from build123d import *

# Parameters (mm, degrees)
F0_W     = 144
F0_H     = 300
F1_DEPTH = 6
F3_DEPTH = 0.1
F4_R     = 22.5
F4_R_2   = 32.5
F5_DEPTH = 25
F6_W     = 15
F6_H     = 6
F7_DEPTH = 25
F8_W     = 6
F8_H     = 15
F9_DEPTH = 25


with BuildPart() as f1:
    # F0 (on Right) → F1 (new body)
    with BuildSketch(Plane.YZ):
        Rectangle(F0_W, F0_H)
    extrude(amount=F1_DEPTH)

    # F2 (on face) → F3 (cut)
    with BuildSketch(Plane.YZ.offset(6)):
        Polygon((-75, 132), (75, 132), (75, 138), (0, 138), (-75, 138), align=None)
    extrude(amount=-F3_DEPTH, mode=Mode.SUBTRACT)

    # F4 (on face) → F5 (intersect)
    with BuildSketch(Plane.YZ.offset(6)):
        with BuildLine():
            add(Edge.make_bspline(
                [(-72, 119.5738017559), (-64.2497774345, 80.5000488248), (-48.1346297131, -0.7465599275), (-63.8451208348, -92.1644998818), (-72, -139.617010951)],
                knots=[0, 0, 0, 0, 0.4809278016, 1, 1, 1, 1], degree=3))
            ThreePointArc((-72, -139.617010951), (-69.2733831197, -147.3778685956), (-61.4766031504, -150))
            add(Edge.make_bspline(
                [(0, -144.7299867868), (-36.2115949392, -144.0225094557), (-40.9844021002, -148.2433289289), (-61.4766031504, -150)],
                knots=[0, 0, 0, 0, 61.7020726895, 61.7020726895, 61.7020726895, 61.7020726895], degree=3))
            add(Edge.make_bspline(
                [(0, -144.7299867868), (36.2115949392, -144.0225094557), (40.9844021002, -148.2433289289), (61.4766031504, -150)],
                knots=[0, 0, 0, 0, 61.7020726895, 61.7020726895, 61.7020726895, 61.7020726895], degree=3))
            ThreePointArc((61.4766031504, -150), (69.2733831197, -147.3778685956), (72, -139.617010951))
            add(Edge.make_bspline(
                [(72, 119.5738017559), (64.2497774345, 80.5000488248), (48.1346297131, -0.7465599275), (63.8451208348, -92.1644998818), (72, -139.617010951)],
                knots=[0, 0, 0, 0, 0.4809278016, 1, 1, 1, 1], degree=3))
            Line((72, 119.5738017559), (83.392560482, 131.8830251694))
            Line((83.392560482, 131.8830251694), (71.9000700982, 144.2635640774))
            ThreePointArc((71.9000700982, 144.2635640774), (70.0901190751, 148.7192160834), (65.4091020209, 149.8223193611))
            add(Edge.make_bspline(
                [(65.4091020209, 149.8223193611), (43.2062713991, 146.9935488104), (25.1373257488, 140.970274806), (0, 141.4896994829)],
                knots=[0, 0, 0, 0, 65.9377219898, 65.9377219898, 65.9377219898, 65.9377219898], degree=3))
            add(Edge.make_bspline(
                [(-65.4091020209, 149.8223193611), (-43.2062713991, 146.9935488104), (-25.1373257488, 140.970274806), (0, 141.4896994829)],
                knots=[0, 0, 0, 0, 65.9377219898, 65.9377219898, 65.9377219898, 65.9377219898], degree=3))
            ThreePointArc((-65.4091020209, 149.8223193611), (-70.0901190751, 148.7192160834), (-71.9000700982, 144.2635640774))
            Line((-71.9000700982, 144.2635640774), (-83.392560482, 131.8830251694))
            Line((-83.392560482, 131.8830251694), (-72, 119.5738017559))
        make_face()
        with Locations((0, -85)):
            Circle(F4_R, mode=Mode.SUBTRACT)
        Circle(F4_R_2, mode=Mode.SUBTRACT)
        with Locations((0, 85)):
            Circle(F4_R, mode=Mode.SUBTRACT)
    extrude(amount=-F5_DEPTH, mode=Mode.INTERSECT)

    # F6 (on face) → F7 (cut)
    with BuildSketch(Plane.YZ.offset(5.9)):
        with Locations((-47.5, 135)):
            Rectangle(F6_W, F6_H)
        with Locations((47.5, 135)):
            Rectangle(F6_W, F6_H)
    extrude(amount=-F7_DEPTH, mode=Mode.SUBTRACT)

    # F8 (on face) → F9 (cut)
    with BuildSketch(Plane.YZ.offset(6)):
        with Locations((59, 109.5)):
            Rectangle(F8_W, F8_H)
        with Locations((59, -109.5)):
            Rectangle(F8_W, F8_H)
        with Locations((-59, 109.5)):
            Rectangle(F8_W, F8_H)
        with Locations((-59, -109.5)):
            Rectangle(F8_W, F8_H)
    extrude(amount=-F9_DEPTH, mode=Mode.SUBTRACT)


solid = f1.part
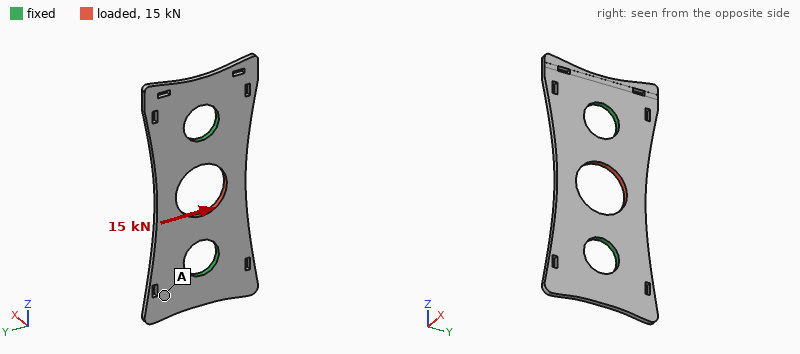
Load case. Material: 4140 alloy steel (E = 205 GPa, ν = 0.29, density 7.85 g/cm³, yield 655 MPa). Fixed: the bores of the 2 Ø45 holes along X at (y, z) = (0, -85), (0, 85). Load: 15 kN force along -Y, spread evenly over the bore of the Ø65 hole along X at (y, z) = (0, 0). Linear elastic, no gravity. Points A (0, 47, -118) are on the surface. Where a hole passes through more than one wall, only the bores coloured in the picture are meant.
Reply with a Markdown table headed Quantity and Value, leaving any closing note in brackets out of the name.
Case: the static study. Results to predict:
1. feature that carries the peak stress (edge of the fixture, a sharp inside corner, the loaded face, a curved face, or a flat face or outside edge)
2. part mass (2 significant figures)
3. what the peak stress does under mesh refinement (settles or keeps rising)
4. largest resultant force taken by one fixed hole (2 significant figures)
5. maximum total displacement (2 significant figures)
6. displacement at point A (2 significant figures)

| Quantity | Value |
|---|---|
| feature that carries the peak stress | edge of the fixture |
| part mass | 1.4 kg |
| what the peak stress does under mesh refinement | keeps rising |
| largest resultant force taken by one fixed hole | 7.5 kN |
| maximum total displacement | 14 µm |
| displacement at point A | 2.2 µm |
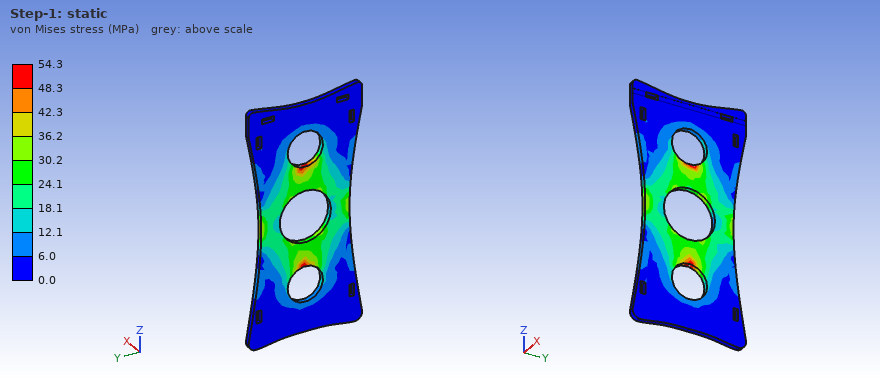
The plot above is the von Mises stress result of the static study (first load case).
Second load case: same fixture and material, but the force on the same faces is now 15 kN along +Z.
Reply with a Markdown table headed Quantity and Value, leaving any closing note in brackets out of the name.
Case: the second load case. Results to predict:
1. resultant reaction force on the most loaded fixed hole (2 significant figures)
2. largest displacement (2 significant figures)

| Quantity | Value |
|---|---|
| resultant reaction force on the most loaded fixed hole | 7.5 kN |
| largest displacement | 5.2 µm |
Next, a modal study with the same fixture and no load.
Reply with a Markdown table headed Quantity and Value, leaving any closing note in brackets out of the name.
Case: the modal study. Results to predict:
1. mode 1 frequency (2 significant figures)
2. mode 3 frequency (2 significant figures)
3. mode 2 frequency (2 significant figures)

| Quantity | Value |
|---|---|
| mode 1 frequency | 1400 Hz |
| mode 3 frequency | 1500 Hz |
| mode 2 frequency | 1500 Hz |
